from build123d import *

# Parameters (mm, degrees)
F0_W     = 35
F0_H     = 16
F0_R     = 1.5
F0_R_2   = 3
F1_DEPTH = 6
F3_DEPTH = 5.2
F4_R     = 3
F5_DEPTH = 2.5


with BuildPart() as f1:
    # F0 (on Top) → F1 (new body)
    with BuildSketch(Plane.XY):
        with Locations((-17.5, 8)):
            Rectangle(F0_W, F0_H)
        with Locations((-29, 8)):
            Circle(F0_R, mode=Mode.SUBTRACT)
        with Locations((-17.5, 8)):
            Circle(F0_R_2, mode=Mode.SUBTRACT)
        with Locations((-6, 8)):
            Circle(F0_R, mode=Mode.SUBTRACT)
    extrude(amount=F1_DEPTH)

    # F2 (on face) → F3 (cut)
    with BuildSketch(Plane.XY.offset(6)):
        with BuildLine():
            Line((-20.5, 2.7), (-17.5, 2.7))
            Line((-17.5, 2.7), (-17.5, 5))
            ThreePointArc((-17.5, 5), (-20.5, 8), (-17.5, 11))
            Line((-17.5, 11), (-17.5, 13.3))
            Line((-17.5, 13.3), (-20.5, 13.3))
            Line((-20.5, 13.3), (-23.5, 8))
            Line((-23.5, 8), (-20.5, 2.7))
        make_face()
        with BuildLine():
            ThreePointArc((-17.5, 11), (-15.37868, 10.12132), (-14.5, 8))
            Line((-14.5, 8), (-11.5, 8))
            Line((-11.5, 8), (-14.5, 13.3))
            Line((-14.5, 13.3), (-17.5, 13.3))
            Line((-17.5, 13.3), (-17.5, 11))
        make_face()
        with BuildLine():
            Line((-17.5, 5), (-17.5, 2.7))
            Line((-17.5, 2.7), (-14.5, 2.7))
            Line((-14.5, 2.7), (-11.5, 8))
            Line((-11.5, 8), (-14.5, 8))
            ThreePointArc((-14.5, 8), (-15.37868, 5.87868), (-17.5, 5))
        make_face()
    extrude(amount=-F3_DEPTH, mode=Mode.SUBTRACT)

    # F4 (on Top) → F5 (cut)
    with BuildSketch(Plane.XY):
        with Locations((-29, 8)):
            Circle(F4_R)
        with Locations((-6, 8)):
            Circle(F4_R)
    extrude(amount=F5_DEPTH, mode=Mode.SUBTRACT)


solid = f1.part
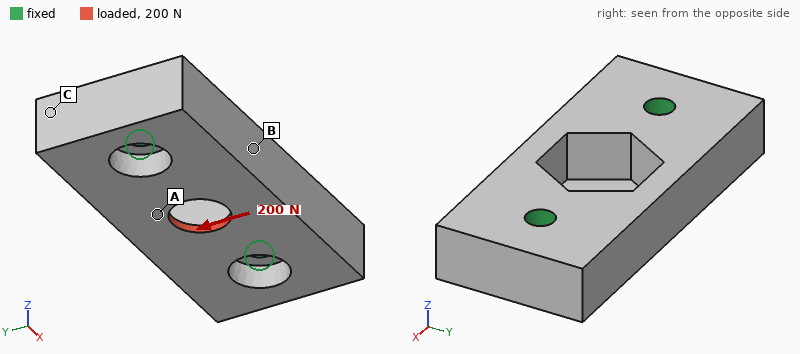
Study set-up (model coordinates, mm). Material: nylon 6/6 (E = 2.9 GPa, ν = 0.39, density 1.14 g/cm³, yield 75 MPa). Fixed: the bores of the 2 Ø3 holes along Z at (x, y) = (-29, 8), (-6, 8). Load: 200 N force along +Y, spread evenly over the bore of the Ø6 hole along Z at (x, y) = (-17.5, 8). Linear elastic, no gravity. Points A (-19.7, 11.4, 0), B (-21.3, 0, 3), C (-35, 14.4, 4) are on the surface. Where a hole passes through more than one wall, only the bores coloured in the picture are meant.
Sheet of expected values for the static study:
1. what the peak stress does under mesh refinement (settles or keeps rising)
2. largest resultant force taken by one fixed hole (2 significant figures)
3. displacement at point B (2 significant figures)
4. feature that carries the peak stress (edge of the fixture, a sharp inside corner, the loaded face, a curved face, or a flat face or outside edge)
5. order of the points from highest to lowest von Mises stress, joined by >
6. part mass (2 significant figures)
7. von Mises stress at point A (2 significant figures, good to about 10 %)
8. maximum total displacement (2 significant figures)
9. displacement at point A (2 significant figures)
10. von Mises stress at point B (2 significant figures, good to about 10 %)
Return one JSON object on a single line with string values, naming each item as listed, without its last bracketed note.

{"what the peak stress does under mesh refinement": "keeps rising", "largest resultant force taken by one fixed hole": "100 N", "displacement at point B": "51 µm", "feature that carries the peak stress": "edge of the fixture", "order of the points from highest to lowest von Mises stress, joined by >": "A > B > C", "part mass": "3.0 g", "von Mises stress at point A": "12 MPa", "maximum total displacement": "77 µm", "displacement at point A": "60 µm", "von Mises stress at point B": "4.7 MPa"}
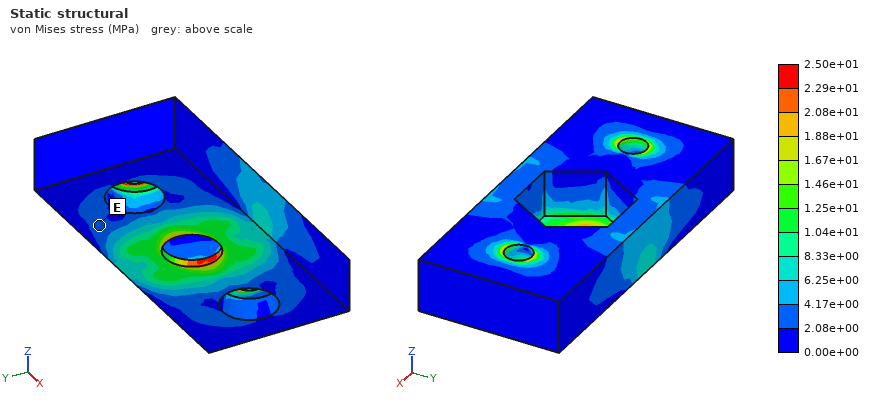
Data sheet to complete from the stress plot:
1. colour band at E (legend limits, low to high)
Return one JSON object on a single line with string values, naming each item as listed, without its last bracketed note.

{"colour band at E": "2.08e+00 to 4.17e+00 MPa"}
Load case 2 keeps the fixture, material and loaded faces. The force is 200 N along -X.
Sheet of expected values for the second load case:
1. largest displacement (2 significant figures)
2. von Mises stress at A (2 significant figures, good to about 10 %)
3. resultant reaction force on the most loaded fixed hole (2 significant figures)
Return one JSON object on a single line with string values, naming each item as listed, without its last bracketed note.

{"largest displacement": "38 µm", "von Mises stress at A": "10 MPa", "resultant reaction force on the most loaded fixed hole": "100 N"}
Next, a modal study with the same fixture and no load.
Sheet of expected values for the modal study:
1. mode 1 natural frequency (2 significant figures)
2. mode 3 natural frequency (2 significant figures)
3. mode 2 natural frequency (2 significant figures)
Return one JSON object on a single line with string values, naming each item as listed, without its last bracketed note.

{"mode 1 natural frequency": "7100 Hz", "mode 3 natural frequency": "10 kHz", "mode 2 natural frequency": "9900 Hz"}
